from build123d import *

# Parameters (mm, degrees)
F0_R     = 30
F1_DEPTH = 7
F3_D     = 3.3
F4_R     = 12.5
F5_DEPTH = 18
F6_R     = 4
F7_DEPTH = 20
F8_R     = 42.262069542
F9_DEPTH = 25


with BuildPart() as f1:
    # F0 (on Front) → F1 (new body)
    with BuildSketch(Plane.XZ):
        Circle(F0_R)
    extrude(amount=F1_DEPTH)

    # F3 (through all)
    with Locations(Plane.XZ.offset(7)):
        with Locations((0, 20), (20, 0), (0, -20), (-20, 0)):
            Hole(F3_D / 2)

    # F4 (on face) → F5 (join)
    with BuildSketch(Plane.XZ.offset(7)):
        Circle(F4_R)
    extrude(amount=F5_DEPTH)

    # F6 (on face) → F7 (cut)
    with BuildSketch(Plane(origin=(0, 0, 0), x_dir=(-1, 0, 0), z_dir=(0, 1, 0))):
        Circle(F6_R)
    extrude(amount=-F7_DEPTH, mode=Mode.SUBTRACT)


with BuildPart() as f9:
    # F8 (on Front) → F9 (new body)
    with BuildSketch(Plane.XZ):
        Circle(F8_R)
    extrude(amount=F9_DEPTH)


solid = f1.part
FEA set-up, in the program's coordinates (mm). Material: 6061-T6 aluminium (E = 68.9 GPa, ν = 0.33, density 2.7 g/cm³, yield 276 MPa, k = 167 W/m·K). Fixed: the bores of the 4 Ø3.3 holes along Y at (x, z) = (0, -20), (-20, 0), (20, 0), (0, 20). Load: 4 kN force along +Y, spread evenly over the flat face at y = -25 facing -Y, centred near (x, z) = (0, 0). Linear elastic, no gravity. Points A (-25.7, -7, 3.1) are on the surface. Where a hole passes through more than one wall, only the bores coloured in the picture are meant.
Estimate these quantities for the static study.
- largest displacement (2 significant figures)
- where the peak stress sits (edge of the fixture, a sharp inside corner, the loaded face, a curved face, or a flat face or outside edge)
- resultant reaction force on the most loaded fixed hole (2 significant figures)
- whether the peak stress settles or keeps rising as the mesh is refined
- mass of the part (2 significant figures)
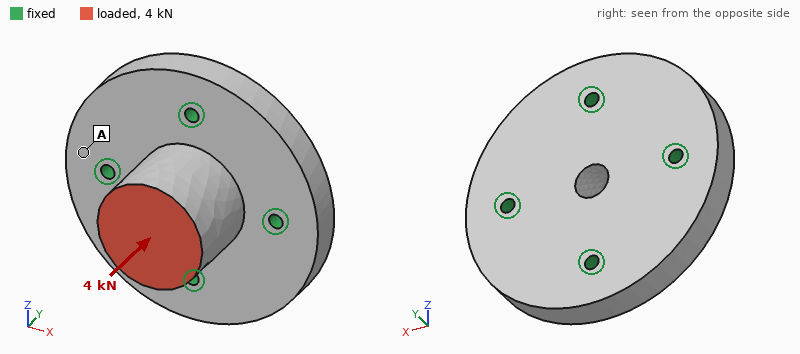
9.8 µm
edge of the fixture
1.0 kN
keeps rising
74 g
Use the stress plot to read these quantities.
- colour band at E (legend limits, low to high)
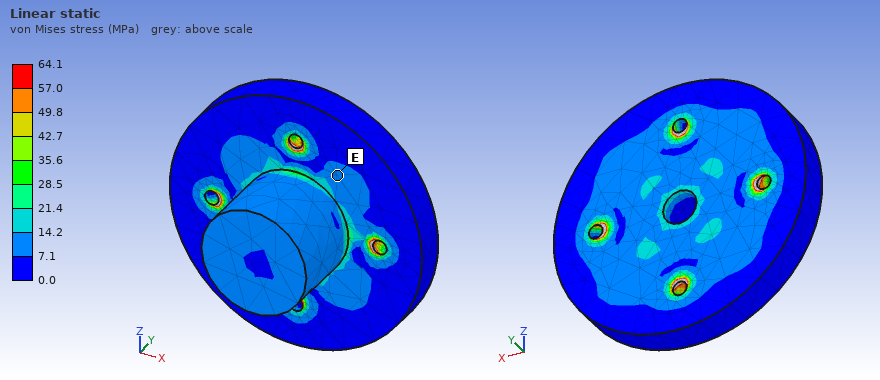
7.1 to 14.2 MPa
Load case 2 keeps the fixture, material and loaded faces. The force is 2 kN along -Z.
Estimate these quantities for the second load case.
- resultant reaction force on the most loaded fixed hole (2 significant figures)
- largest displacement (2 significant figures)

1.3 kN
21 µm
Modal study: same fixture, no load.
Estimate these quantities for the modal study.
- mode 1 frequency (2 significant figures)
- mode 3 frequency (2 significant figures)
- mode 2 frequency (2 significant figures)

16 kHz
18 kHz
16 kHz
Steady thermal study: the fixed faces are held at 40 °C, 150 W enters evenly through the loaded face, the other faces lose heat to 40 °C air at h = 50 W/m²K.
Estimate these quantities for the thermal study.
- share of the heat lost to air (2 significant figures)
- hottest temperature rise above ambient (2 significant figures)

4.0 %
59 K
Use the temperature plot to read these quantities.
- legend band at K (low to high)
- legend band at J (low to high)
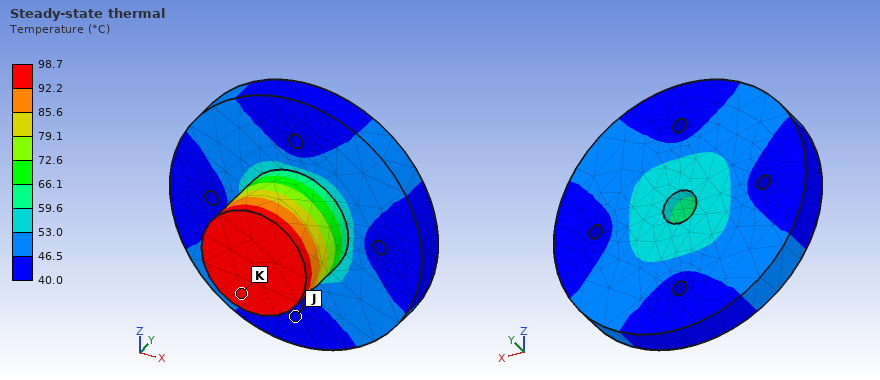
92.2 to 98.7 °C
40.0 to 46.5 °C
